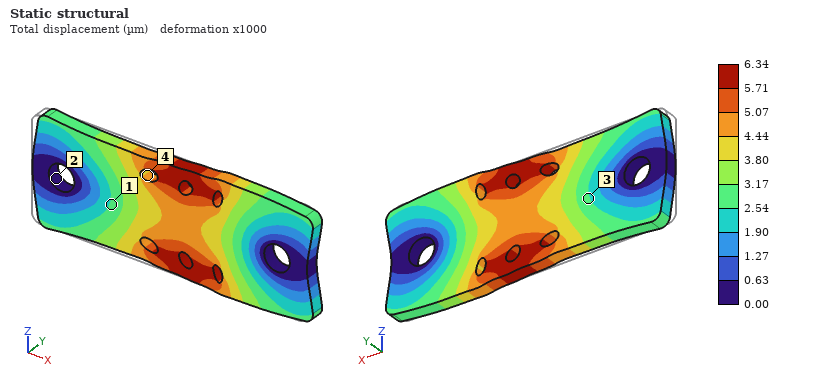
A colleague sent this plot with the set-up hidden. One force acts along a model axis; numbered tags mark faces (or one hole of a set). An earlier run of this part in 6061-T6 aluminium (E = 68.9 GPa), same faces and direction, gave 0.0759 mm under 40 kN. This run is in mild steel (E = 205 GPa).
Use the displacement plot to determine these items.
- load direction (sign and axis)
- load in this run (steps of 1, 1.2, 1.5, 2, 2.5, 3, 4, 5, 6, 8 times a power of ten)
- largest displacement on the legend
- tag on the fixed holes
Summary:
+X
10 kN
6.34 µm
2
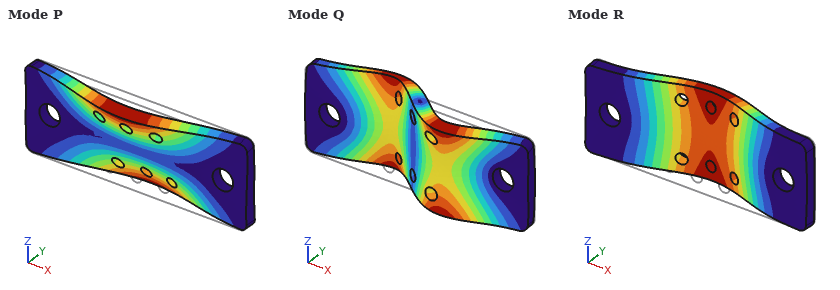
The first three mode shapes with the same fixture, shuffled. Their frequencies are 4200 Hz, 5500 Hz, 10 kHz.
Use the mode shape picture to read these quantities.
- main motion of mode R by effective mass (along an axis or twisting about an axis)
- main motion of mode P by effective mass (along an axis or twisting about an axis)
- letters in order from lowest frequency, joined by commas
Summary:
along Y
twisting about X
R, P, Q
